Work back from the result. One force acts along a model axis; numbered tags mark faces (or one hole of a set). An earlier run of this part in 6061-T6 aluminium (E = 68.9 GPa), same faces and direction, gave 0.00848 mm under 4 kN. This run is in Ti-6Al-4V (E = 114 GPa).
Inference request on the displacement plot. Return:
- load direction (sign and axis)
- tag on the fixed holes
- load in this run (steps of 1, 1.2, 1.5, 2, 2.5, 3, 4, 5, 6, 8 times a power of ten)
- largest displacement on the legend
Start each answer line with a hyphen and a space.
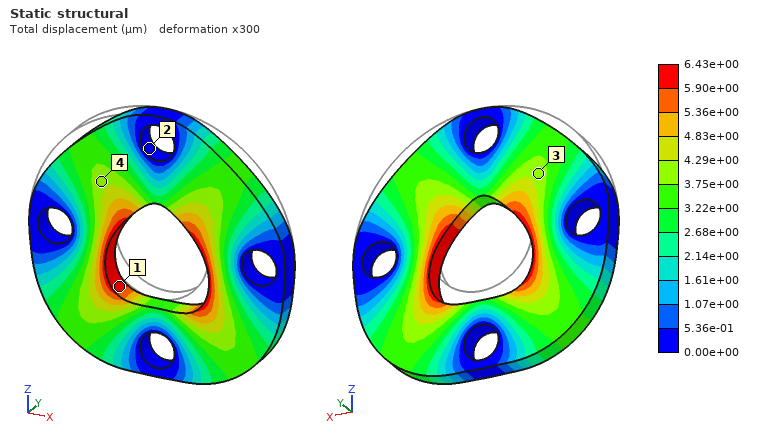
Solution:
- -Z
- 2
- 5 kN
- 6.43e+00 µm
